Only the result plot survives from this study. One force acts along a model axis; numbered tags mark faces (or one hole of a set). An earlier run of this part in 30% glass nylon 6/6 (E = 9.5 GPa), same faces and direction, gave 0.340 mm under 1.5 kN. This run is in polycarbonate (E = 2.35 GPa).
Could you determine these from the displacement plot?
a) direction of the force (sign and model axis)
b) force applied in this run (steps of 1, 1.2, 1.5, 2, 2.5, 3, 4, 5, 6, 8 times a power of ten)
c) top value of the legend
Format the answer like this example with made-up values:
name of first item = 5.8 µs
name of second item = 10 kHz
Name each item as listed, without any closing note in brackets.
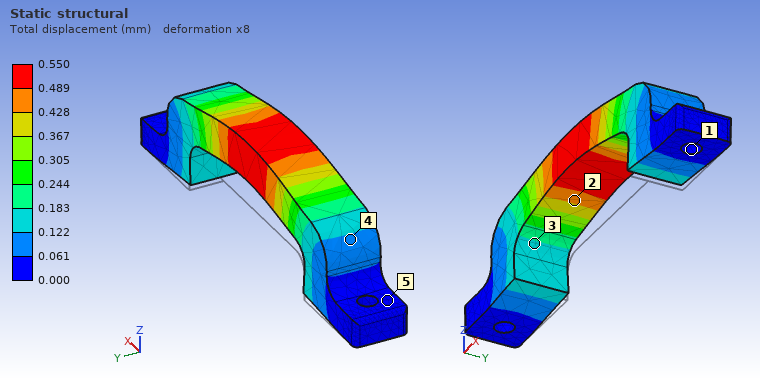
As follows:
direction of the force = +Z
force applied in this run = 600 N
top value of the legend = 0.550 mm
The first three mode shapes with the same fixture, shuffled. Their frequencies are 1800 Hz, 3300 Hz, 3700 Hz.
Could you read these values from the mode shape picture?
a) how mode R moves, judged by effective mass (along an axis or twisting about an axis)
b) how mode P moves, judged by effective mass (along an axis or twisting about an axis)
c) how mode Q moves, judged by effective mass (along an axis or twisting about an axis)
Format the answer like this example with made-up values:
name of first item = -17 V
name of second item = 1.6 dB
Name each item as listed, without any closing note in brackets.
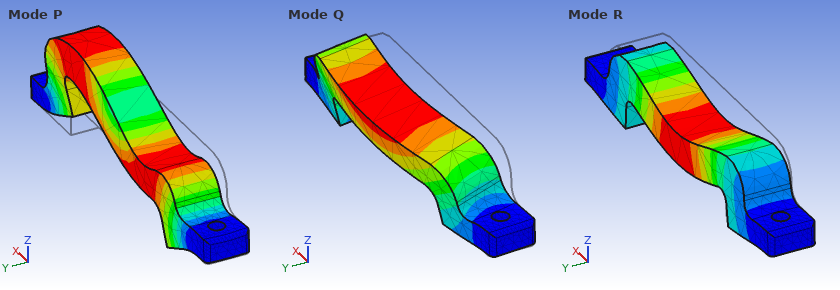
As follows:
how mode R moves, judged by effective mass = along Z
how mode P moves, judged by effective mass = along X
how mode Q moves, judged by effective mass = along Y
